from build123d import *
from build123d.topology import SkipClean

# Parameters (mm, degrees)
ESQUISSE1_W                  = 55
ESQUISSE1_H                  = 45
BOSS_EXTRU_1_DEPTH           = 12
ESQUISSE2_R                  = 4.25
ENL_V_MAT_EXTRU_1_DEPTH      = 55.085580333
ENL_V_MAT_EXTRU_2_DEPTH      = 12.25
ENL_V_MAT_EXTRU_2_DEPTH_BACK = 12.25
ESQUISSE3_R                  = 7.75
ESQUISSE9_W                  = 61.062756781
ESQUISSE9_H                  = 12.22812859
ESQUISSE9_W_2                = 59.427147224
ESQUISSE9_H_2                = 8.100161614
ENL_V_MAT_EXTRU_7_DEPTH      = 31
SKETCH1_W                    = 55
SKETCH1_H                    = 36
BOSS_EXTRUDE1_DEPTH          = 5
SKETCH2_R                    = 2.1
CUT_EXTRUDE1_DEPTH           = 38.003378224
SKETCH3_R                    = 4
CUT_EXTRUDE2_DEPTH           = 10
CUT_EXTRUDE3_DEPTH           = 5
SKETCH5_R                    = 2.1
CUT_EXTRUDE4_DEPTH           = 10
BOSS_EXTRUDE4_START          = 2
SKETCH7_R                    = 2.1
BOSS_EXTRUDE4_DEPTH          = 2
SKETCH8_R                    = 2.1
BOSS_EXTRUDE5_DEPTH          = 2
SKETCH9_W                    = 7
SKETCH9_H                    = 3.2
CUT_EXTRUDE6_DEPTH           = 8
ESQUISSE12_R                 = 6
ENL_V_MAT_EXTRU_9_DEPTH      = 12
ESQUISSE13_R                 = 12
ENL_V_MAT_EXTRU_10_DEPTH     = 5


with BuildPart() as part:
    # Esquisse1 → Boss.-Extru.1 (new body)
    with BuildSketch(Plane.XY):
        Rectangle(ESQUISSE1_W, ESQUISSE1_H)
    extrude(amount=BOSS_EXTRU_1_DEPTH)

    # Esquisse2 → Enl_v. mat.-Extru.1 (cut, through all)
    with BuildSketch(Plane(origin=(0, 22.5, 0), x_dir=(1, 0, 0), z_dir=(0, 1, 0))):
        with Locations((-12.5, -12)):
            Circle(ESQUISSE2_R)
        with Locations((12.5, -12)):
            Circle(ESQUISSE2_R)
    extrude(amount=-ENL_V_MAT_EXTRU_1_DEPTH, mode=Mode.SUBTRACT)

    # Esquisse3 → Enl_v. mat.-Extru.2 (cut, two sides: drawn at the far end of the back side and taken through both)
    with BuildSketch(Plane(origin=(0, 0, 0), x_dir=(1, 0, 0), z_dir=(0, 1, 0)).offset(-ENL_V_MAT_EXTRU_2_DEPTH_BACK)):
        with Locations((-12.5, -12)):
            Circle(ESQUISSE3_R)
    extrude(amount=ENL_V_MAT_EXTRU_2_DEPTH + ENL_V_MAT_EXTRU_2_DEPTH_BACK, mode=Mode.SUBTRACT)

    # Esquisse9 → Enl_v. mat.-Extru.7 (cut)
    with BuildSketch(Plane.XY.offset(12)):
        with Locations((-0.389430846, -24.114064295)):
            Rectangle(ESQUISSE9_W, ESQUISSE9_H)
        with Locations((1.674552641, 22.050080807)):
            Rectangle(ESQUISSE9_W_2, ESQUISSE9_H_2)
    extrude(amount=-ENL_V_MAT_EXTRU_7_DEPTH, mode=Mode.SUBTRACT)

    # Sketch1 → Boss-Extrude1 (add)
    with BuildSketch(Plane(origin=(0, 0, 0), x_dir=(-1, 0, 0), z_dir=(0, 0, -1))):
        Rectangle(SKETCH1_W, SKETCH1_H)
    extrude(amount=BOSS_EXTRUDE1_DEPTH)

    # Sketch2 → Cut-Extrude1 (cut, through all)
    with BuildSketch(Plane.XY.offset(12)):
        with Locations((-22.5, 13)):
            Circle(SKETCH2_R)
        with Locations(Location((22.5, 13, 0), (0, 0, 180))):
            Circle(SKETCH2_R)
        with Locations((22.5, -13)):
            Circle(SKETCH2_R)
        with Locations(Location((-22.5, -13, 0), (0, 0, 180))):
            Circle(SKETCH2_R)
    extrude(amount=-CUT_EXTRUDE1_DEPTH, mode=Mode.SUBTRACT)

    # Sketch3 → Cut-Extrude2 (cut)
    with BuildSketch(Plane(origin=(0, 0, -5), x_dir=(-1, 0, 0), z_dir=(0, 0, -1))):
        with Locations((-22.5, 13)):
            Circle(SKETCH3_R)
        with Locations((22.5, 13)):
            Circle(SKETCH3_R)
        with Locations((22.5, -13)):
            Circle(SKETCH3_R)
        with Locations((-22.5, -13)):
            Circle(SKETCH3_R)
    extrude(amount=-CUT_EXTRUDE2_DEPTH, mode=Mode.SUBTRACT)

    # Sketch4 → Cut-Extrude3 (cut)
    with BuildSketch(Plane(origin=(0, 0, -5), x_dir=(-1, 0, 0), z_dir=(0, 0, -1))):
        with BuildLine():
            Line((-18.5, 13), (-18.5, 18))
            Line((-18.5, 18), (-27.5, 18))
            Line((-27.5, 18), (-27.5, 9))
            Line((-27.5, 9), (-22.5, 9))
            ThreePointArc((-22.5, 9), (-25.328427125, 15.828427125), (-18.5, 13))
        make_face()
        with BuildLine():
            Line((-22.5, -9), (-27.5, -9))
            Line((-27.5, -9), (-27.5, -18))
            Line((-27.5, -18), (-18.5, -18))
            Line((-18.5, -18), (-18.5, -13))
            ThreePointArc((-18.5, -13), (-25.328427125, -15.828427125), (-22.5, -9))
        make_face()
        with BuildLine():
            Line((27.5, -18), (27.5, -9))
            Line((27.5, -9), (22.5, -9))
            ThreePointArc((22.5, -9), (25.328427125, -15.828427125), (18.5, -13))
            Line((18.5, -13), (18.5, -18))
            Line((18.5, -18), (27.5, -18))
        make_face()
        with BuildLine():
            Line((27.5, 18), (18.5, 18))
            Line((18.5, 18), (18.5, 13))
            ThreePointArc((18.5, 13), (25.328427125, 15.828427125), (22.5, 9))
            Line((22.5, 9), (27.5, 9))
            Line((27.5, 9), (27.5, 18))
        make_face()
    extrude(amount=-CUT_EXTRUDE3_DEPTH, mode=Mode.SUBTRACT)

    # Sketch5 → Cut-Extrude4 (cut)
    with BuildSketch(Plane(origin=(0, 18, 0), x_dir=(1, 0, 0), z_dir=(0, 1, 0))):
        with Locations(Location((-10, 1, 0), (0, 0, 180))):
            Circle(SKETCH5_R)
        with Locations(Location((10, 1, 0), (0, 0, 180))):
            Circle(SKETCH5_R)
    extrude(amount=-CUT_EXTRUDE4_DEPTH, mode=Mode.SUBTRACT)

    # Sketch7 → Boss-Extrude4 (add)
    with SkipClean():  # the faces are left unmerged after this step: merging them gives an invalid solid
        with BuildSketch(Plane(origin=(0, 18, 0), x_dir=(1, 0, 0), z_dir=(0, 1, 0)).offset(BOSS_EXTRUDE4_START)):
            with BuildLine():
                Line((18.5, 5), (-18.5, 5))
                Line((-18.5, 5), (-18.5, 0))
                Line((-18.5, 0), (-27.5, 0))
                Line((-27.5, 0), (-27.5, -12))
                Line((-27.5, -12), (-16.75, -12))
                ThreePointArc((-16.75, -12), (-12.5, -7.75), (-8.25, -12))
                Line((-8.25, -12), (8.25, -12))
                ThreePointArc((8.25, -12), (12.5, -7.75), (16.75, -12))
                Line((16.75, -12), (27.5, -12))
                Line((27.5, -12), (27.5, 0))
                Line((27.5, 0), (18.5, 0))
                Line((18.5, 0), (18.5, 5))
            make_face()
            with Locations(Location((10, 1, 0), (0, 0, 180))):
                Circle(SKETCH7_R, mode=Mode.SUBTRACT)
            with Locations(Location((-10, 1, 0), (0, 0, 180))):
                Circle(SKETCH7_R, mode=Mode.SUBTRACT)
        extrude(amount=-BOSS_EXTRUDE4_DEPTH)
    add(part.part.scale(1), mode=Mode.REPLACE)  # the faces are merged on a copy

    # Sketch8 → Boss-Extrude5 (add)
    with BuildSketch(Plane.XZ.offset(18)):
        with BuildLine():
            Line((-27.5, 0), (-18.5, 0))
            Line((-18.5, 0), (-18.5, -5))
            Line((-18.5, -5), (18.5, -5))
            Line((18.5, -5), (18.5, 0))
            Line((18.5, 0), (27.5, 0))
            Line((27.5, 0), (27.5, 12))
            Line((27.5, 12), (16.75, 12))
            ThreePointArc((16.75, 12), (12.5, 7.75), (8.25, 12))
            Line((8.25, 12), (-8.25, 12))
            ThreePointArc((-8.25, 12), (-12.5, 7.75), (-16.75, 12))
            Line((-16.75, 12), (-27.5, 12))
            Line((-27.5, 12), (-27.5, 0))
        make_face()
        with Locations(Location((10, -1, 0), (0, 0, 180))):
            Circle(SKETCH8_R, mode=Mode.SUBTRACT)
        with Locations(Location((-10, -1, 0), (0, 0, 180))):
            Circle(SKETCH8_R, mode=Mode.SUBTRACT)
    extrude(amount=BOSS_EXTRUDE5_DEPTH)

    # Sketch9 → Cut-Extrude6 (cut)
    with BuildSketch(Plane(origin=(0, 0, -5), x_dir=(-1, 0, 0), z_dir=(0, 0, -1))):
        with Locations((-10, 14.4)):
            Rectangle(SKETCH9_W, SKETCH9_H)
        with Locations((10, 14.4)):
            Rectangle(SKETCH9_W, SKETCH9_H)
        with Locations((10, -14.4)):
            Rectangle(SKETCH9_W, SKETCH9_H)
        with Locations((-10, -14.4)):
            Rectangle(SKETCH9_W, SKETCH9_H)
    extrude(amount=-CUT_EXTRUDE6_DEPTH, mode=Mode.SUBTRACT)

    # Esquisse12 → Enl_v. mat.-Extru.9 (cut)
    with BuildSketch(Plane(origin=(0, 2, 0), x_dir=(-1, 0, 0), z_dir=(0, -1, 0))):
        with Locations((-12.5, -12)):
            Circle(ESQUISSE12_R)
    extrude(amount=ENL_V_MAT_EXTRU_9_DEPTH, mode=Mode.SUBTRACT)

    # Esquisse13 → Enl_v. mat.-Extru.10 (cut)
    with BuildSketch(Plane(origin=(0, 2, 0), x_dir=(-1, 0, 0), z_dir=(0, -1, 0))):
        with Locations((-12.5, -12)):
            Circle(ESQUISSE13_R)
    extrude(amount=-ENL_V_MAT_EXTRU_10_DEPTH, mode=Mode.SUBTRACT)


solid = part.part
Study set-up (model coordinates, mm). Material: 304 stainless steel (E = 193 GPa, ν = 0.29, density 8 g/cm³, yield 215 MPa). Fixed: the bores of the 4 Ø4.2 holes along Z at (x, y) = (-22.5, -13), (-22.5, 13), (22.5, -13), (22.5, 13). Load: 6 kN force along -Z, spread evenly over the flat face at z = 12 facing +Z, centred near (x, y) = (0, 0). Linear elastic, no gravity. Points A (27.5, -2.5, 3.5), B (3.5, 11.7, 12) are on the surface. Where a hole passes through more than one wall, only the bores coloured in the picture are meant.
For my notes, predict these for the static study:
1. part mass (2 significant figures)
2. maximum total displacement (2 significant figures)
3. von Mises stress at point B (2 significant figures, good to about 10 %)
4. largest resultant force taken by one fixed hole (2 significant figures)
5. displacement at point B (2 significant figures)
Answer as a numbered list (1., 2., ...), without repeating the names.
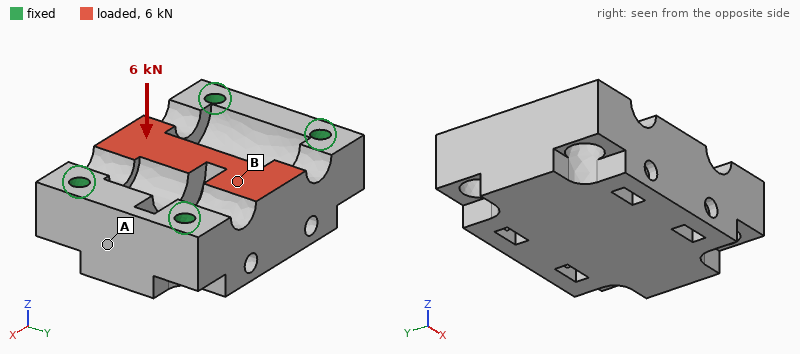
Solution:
1. 220 g
2. 6.0 µm
3. 15 MPa
4. 2.0 kN
5. 5.3 µm
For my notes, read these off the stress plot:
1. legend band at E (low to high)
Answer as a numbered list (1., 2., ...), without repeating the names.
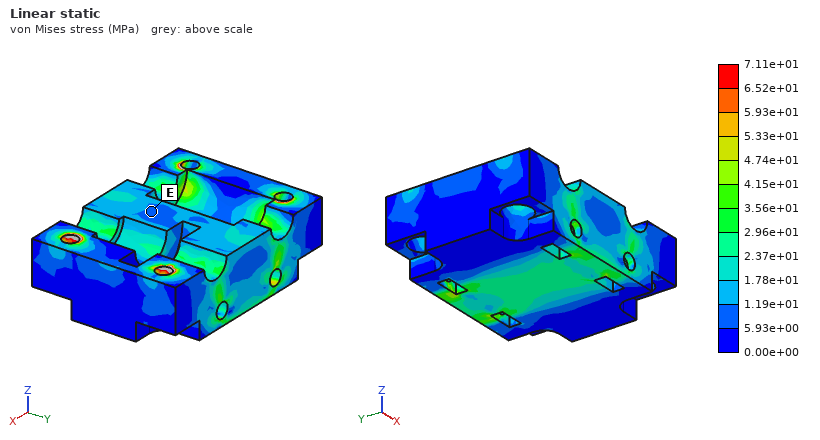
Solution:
1. 5.93e+00 to 1.19e+01 MPa
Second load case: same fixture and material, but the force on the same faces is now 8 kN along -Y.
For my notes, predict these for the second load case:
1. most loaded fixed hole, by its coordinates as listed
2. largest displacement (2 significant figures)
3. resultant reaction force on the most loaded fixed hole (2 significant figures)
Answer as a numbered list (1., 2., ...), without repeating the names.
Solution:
1. (22.5, -13)
2. 15 µm
3. 2.4 kN
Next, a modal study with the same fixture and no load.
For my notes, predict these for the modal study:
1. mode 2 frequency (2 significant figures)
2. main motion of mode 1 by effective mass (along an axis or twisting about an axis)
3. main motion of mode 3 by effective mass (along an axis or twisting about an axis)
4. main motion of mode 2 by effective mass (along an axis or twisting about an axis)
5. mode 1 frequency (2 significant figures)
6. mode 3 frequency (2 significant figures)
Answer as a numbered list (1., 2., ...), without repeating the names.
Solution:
1. 18 kHz
2. along Z
3. along Y
4. along Y
5. 17 kHz
6. 19 kHz
